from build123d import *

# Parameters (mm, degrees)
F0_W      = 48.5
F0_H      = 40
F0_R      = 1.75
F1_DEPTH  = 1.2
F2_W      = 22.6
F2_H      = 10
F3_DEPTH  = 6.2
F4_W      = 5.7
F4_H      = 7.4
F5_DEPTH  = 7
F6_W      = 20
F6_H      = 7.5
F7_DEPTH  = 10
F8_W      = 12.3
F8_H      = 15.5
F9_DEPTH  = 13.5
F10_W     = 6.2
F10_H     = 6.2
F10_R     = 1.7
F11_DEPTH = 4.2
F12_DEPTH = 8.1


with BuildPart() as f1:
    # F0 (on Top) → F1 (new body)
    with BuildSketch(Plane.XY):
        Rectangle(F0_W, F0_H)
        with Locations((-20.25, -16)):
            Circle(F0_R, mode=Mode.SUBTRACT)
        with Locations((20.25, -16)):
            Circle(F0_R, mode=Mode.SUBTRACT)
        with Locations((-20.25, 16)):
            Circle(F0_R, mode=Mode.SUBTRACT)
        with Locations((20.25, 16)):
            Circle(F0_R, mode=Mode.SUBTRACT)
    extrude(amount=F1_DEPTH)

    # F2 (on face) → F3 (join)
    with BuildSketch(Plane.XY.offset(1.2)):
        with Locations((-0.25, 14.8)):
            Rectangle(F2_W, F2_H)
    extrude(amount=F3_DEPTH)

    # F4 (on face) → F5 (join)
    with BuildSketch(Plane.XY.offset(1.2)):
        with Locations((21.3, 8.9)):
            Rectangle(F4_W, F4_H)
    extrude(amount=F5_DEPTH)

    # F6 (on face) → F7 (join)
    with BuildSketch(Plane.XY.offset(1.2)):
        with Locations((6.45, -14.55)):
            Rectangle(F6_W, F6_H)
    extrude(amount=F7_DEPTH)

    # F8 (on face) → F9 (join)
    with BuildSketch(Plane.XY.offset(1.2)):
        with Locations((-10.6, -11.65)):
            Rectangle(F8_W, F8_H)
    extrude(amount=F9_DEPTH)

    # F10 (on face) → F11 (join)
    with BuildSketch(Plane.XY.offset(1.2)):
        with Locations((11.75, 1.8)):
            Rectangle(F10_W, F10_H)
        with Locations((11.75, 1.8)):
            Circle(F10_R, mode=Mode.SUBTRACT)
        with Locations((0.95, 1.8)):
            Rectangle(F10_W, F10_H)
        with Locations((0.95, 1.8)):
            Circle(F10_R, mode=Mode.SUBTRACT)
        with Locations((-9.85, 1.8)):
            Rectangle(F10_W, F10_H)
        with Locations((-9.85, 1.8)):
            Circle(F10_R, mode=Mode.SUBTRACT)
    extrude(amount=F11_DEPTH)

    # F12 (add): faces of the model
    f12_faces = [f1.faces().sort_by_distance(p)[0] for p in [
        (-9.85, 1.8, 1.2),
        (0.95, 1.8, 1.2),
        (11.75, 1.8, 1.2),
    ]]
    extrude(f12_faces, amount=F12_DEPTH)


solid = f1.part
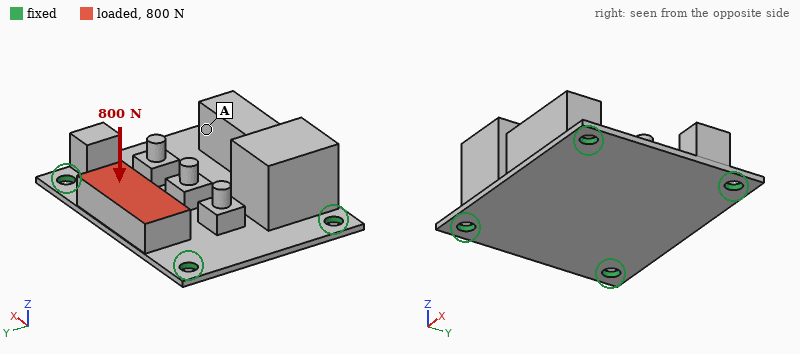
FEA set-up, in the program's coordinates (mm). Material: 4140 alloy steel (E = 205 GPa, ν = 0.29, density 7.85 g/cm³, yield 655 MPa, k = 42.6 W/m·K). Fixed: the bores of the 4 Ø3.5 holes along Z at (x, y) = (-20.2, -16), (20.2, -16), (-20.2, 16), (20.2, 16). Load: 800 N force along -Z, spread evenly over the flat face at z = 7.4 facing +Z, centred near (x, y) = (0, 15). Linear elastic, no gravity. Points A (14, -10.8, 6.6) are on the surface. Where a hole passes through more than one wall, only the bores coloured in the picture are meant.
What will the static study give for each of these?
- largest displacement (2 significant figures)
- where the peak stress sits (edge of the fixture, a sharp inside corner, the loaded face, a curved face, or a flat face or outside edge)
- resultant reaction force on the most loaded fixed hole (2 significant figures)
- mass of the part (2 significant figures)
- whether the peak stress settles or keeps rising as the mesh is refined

69 µm
edge of the fixture
480 N
68 g
keeps rising
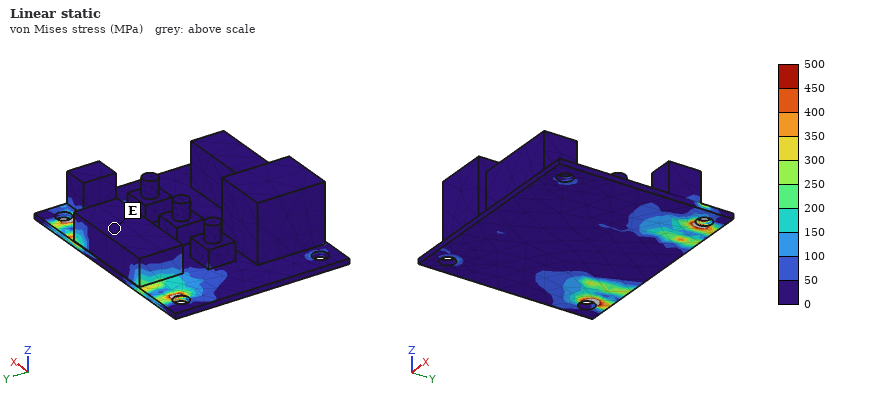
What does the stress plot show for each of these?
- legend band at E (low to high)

0 to 50 MPa
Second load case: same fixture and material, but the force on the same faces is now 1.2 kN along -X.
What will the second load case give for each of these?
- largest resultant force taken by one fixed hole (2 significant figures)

550 N
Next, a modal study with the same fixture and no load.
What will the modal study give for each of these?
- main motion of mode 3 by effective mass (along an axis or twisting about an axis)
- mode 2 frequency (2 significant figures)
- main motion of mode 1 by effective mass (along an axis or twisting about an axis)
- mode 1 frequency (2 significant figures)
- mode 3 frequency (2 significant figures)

along Z
3200 Hz
along Z
2500 Hz
4900 Hz
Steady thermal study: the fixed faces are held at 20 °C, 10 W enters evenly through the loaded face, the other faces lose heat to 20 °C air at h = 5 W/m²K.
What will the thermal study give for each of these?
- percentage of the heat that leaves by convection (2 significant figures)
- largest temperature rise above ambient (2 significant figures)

6.3 %
60 K
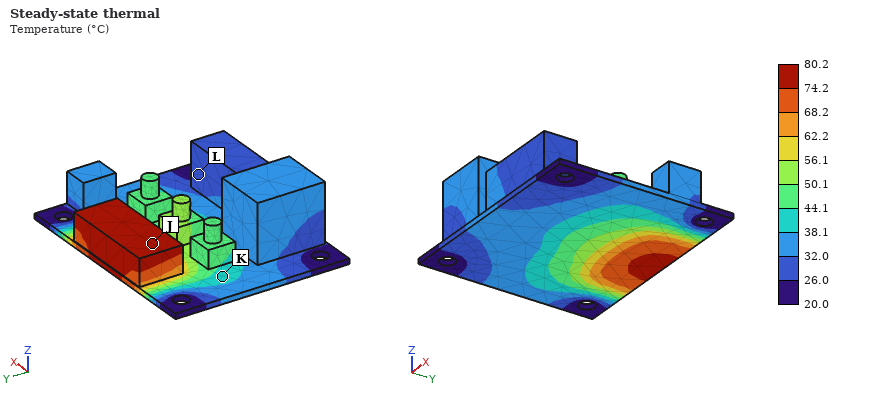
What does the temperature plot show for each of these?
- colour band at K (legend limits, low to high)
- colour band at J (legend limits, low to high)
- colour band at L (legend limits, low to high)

38.1 to 44.1 °C
74.2 to 80.2 °C
26.0 to 32.0 °C
